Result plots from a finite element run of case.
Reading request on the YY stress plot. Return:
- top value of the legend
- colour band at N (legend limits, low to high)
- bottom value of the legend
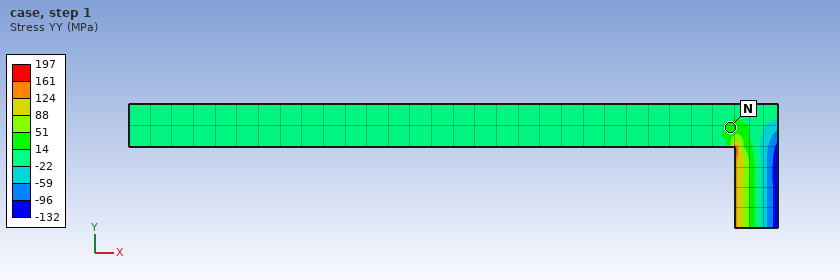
197 MPa
14 to 51 MPa
-132 MPa
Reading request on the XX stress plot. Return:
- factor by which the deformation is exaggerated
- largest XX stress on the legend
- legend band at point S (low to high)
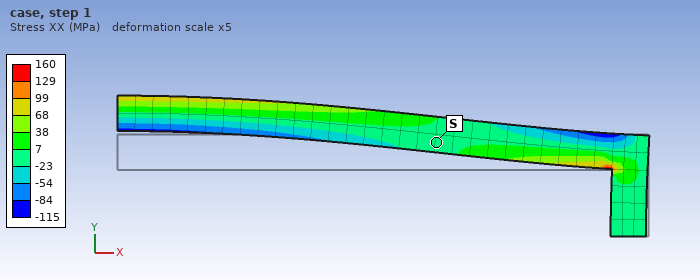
5
160 MPa
-23 to 7 MPa
